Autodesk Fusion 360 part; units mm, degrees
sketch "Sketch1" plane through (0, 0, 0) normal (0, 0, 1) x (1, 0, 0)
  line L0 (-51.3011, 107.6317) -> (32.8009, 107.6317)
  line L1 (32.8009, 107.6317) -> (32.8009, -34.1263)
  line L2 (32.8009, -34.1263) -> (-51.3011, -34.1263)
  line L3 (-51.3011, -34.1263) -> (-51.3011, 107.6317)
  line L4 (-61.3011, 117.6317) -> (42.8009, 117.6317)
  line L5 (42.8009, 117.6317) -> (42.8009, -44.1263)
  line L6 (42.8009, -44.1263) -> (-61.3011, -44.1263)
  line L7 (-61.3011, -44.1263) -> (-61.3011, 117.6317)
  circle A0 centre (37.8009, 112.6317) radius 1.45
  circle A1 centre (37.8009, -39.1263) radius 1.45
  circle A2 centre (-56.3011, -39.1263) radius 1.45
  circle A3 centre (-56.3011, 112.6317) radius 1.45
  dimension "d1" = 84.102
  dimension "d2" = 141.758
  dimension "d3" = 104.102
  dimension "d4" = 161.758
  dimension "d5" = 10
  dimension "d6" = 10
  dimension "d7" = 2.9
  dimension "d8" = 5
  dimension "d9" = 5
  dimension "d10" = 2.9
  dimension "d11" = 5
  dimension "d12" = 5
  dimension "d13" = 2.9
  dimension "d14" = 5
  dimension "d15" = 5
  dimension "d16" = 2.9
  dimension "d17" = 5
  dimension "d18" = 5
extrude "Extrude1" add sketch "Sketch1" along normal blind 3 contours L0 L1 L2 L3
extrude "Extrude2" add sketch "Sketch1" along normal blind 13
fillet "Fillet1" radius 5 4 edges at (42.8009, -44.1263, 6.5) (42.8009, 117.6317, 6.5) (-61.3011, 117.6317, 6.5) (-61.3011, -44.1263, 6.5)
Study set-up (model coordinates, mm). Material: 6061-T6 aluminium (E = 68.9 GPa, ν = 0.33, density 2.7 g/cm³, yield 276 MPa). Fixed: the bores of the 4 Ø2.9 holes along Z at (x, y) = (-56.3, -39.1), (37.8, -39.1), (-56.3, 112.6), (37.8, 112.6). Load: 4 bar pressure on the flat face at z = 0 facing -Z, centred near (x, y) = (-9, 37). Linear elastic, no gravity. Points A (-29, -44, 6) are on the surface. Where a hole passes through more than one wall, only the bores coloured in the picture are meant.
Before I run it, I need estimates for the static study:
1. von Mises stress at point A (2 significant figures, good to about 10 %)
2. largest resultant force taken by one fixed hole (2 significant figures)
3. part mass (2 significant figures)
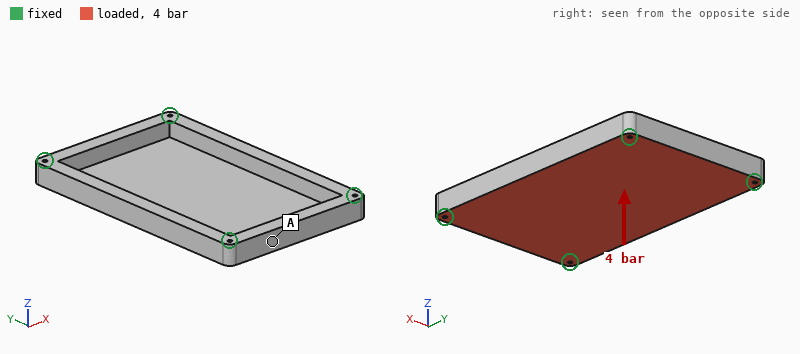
13 MPa
2.2 kN
270 g
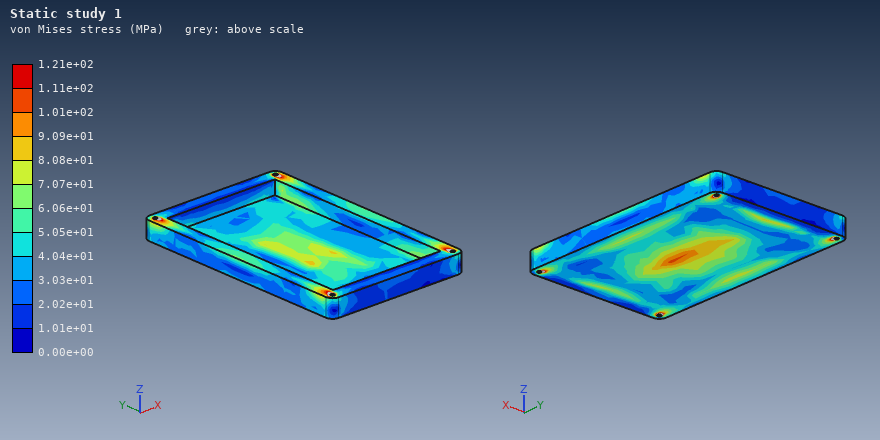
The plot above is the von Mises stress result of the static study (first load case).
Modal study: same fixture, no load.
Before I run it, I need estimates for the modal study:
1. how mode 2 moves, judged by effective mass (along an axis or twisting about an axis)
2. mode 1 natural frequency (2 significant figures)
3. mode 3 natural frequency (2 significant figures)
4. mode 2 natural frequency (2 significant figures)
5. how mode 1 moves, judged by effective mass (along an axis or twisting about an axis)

twisting about Y
1800 Hz
3300 Hz
2600 Hz
along Z
